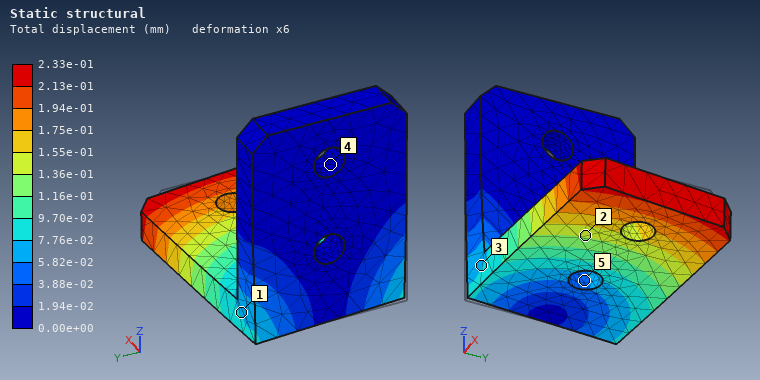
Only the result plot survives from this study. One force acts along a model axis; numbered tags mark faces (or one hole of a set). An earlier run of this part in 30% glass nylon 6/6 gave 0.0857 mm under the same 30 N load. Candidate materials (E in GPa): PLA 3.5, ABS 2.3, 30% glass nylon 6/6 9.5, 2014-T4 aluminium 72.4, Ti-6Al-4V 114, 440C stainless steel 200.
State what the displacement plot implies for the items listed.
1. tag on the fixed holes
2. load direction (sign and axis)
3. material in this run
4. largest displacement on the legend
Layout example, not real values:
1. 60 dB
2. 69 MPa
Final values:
1. 4
2. +Y
3. PLA
4. 2.33e-01 mm
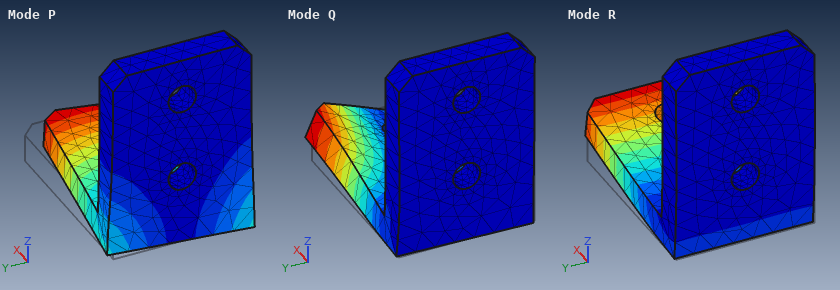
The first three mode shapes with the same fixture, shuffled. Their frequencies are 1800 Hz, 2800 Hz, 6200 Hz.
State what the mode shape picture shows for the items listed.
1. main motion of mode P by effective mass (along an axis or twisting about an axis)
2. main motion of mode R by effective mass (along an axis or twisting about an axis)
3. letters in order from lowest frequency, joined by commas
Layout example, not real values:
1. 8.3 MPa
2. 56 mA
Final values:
1. along Y
2. along Z
3. R, P, Q
